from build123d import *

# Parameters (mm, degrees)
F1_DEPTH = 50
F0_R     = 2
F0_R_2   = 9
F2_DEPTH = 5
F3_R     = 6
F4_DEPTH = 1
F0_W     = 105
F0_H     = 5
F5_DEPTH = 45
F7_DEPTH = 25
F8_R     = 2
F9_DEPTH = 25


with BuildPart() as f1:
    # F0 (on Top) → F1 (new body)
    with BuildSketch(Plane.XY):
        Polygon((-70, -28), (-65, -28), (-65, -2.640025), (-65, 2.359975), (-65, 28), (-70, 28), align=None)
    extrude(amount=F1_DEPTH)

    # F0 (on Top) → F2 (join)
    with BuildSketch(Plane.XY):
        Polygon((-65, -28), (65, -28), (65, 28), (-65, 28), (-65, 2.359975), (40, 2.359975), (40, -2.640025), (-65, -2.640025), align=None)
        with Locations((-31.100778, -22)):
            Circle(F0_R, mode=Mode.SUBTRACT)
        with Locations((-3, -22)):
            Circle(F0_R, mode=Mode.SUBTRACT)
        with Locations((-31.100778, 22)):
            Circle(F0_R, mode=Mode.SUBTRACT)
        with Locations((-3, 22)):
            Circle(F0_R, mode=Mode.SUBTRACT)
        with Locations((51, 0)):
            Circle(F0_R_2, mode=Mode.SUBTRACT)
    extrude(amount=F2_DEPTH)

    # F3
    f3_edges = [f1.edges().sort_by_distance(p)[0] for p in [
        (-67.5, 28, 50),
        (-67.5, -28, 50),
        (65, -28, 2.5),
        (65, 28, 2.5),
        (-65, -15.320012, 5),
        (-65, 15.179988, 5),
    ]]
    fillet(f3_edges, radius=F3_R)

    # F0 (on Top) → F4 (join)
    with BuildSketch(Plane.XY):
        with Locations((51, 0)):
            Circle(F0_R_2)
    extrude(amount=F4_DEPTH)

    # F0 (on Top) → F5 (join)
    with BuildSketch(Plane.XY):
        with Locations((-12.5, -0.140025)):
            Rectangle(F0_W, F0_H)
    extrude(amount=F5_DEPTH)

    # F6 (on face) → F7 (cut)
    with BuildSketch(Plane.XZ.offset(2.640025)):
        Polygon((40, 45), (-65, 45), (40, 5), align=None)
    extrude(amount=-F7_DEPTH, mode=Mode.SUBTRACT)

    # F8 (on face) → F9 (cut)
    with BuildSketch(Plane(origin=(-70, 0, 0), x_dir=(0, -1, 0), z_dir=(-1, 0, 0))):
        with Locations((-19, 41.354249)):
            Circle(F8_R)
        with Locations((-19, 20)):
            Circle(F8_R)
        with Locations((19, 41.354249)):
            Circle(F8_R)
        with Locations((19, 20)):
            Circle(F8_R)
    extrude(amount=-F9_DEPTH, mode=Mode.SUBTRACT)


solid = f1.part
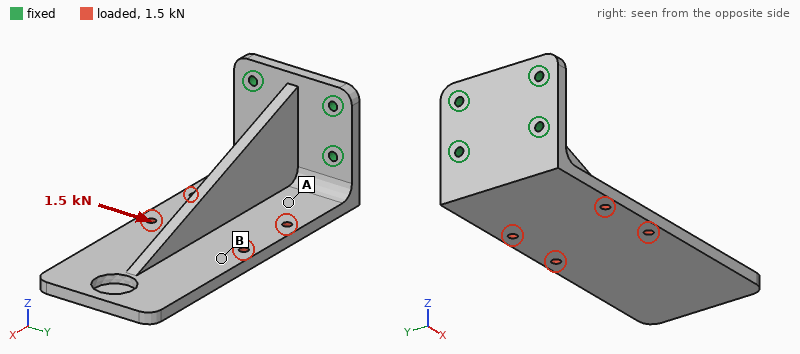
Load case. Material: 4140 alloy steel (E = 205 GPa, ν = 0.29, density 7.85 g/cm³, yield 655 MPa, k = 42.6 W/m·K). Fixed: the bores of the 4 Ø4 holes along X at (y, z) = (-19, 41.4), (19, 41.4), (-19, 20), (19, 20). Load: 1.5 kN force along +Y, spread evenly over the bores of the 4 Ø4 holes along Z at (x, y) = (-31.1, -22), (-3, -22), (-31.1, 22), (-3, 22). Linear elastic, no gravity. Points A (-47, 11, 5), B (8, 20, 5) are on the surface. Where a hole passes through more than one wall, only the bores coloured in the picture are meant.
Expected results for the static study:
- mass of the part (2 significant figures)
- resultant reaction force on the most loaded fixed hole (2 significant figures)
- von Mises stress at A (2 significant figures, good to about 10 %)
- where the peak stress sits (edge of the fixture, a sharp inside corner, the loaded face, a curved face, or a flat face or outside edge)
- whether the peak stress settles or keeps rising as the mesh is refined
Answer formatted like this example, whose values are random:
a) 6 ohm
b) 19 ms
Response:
a) 470 g
b) 2.2 kN
c) 18 MPa
d) edge of the fixture
e) keeps rising
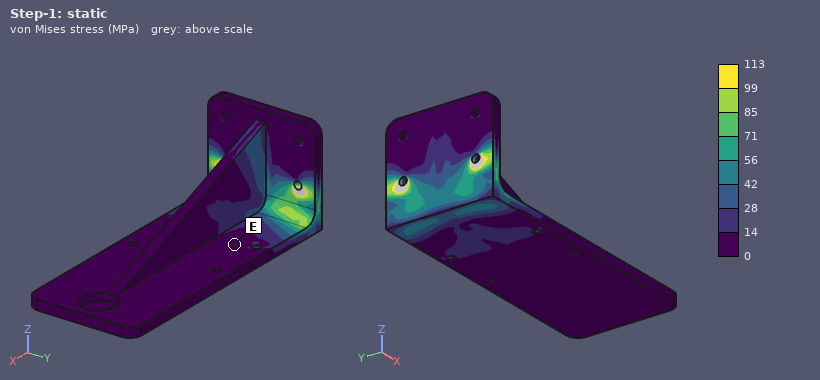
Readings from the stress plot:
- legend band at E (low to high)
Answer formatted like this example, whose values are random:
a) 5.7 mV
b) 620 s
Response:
a) 0 to 14 MPa
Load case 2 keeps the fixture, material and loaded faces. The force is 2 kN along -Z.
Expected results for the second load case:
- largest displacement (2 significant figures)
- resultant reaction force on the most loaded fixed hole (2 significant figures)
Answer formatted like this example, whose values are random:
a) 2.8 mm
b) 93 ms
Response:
a) 0.23 mm
b) 1.8 kN
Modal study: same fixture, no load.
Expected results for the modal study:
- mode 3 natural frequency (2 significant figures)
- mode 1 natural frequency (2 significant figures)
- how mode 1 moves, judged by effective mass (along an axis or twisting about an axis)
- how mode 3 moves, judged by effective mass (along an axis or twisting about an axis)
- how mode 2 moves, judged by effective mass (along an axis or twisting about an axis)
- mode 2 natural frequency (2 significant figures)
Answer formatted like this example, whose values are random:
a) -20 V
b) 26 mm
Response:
a) 1400 Hz
b) 810 Hz
c) along Z
d) twisting about X
e) along Y
f) 870 Hz
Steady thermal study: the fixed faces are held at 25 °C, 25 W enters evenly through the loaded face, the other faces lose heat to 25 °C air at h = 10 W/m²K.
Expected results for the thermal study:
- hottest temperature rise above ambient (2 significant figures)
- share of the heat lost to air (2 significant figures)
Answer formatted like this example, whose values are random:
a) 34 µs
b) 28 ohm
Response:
a) 71 K
b) 39 %
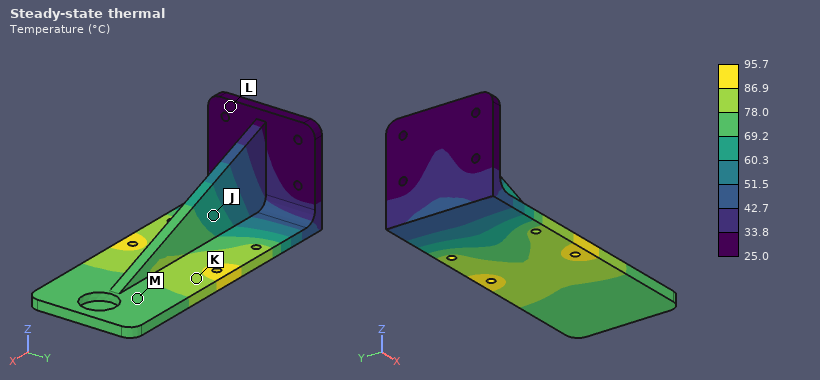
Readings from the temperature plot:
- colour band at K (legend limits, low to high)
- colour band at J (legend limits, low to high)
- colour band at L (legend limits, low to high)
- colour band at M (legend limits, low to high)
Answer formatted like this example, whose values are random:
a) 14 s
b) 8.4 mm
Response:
a) 78.0 to 86.9 °C
b) 60.3 to 69.2 °C
c) 25.0 to 33.8 °C
d) 69.2 to 78.0 °C
